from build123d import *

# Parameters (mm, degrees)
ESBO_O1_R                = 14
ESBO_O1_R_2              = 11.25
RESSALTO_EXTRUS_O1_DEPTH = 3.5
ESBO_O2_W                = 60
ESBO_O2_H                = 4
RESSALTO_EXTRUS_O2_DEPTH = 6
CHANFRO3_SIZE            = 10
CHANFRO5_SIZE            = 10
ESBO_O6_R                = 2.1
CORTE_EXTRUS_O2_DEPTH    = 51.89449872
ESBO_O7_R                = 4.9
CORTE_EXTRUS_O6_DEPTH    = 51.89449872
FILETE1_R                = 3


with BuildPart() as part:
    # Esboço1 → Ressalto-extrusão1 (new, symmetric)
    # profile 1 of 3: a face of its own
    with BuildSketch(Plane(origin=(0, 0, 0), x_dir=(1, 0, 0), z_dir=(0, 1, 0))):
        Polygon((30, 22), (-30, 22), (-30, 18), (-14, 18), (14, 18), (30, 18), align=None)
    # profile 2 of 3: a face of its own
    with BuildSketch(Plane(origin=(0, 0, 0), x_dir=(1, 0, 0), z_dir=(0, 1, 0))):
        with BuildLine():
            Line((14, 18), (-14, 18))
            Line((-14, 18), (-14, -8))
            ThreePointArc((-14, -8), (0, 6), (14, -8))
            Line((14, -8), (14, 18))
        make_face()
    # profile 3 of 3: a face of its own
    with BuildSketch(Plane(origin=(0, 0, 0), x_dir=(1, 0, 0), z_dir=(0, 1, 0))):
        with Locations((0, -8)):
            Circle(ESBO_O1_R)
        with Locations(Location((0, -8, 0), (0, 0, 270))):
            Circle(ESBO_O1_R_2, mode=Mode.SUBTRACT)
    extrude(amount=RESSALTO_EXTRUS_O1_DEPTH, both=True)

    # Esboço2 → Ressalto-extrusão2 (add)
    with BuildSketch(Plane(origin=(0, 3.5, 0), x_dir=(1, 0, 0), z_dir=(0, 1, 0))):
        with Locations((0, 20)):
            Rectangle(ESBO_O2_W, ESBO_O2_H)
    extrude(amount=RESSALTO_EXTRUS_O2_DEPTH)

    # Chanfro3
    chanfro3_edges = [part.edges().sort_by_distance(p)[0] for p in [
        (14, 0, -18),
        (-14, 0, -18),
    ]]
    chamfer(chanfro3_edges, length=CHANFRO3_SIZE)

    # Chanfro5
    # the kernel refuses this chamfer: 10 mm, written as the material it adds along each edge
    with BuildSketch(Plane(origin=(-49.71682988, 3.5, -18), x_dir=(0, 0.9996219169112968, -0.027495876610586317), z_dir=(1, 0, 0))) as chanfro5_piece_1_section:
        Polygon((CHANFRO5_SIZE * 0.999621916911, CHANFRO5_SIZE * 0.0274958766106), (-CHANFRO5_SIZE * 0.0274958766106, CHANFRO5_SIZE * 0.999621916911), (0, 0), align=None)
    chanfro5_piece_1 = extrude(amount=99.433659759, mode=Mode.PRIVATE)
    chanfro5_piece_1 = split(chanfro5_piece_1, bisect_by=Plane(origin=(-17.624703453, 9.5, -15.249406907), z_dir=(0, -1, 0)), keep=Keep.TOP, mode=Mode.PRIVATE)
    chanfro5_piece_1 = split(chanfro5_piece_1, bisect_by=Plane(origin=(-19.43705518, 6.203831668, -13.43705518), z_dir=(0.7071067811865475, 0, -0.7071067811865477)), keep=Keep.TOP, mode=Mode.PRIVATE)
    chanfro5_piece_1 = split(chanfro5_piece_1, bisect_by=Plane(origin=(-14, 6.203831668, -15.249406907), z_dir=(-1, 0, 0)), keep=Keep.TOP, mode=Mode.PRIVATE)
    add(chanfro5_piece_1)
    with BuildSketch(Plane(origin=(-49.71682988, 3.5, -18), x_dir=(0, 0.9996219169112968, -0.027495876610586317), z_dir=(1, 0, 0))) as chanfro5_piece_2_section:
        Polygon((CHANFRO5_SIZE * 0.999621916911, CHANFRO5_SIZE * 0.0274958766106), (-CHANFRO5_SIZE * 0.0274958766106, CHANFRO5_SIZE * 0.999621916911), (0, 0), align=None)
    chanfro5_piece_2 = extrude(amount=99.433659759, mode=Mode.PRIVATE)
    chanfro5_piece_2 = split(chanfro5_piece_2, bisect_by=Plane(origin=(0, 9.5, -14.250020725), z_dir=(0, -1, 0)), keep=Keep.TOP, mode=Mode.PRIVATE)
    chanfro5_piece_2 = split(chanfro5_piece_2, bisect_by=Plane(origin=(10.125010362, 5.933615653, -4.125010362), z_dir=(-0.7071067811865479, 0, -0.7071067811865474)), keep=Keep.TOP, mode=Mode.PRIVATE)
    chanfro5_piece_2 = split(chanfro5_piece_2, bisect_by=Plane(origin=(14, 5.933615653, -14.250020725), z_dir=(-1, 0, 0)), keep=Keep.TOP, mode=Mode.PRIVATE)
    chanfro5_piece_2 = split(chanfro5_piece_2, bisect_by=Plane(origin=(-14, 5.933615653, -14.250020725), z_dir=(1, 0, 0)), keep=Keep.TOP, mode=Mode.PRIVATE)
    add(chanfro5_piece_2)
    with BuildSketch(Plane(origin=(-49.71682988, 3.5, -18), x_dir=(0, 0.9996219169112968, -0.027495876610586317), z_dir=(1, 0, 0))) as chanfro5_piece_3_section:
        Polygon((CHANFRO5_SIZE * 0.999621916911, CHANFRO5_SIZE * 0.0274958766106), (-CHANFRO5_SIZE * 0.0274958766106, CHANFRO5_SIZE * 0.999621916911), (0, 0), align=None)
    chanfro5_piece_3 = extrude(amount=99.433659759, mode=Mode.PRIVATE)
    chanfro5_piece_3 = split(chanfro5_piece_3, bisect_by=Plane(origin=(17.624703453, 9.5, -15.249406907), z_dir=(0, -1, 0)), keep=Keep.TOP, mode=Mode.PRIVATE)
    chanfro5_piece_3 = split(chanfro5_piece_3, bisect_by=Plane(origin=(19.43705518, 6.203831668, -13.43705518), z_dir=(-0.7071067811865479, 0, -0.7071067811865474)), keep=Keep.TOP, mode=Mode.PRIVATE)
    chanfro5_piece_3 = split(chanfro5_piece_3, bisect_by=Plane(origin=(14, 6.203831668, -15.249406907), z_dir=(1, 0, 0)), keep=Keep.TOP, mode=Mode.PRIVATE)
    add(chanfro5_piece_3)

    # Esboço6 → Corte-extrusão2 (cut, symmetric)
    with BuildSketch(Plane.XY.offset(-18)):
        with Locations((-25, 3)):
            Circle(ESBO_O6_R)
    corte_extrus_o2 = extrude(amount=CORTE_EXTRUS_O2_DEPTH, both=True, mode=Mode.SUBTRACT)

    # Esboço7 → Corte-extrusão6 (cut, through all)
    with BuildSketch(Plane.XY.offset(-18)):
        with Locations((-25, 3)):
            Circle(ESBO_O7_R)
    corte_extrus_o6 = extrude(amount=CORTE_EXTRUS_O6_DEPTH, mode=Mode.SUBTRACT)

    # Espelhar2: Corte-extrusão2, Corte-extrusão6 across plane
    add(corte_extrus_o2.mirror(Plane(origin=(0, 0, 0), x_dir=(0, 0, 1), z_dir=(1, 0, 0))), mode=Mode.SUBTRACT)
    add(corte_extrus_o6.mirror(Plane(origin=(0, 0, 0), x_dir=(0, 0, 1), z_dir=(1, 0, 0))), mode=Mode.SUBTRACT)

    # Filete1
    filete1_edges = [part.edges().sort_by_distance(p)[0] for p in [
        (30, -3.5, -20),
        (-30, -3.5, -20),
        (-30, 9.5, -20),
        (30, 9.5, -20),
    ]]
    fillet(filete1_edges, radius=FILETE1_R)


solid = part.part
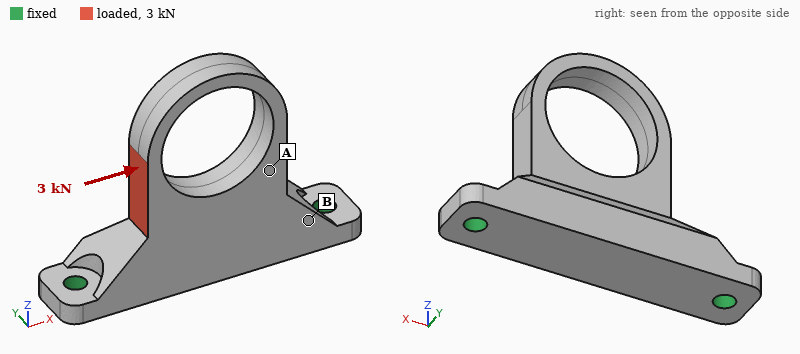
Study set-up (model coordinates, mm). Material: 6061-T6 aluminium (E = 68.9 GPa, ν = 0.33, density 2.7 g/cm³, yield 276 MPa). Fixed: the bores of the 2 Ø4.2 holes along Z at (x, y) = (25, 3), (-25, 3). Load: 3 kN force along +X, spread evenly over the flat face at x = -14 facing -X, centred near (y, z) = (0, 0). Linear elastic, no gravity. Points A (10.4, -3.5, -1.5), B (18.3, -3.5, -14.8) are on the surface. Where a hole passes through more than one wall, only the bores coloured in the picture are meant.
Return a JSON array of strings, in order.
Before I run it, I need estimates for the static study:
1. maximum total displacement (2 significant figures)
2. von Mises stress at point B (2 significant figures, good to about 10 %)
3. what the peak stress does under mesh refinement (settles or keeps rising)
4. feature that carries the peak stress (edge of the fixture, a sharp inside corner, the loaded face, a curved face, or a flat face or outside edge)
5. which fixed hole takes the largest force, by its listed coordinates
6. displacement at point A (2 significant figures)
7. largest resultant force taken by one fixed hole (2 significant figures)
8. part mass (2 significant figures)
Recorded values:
["0.11 mm", "41 MPa", "keeps rising", "edge of the fixture", "(25, 3)", "0.017 mm", "2.2 kN", "26 g"]
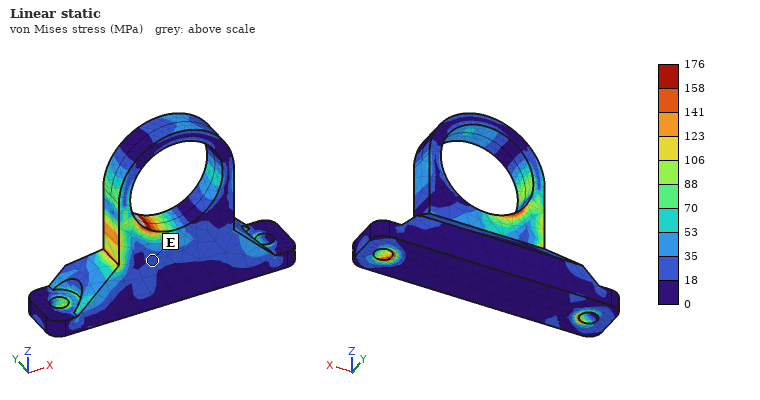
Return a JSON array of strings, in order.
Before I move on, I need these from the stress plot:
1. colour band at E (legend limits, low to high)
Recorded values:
["18 to 35 MPa"]
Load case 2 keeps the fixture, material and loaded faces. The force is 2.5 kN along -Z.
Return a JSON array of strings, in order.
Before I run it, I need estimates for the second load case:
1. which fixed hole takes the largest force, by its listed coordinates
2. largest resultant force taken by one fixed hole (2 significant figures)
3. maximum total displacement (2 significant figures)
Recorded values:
["(-25, 3)", "2.2 kN", "0.12 mm"]
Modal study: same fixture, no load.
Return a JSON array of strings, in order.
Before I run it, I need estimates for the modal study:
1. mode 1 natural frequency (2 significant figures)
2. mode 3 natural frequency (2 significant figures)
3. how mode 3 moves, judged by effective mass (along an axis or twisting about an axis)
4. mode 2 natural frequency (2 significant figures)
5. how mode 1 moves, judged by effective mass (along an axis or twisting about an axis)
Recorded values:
["3500 Hz", "9900 Hz", "along Y", "7500 Hz", "along Y"]
